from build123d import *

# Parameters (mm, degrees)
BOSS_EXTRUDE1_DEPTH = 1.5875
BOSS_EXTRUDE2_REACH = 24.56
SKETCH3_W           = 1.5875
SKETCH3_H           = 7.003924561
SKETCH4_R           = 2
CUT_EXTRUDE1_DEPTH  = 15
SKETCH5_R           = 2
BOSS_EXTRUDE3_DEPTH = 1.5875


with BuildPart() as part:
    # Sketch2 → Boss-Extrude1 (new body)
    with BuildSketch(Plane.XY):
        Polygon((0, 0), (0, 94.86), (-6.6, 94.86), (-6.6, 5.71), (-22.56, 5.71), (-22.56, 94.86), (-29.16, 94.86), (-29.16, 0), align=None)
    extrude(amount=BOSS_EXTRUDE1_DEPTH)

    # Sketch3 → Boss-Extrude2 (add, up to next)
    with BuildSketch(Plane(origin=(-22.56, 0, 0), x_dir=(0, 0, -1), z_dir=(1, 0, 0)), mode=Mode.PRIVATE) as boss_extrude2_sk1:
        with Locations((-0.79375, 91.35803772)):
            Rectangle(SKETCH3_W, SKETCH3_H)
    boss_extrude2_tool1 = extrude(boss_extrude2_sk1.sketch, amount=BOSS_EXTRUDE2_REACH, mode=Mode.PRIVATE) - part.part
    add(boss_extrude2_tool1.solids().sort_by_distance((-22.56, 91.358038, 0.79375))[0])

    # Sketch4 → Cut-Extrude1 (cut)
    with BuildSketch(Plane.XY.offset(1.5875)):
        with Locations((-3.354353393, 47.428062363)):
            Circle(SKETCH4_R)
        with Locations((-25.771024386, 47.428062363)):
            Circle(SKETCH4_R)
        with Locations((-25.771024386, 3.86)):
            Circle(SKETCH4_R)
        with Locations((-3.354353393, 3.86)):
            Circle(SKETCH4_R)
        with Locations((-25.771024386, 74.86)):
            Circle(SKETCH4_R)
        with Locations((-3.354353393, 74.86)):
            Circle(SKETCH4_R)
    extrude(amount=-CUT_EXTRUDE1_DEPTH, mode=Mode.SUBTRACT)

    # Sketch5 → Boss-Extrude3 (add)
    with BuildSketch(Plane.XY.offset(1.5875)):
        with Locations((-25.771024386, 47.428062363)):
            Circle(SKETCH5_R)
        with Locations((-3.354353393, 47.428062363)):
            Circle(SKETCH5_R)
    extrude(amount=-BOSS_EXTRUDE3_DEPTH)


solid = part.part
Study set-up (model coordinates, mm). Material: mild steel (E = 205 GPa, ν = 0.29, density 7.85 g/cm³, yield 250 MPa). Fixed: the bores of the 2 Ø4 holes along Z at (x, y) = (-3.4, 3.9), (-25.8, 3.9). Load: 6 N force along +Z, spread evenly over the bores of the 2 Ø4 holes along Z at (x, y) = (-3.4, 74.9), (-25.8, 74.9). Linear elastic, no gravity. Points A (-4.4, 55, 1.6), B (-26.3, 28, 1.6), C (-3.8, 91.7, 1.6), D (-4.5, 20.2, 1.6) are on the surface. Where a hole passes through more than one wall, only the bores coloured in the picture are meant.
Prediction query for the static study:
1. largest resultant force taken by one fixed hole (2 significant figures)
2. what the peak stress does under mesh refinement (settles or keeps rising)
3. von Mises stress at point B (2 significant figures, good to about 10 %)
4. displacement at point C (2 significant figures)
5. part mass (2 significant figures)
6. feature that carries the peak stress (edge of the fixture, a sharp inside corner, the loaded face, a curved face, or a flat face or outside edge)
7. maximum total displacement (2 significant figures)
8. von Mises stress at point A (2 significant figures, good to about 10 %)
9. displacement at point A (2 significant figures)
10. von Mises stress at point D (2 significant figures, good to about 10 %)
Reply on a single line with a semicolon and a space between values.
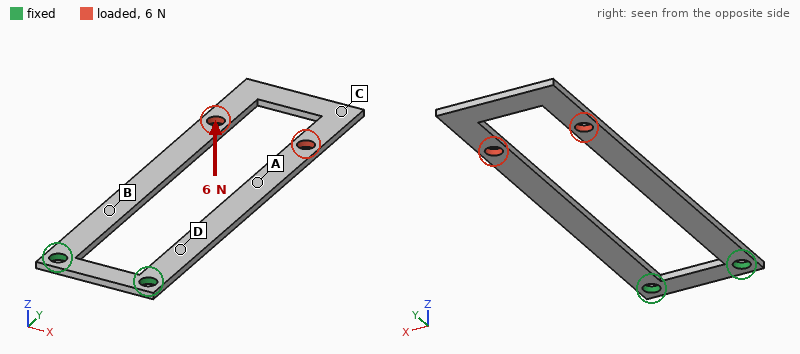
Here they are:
3.0 N; keeps rising; 51 MPa; 1.0 mm; 18 g; edge of the fixture; 1.1 mm; 22 MPa; 0.43 mm; 59 MPa
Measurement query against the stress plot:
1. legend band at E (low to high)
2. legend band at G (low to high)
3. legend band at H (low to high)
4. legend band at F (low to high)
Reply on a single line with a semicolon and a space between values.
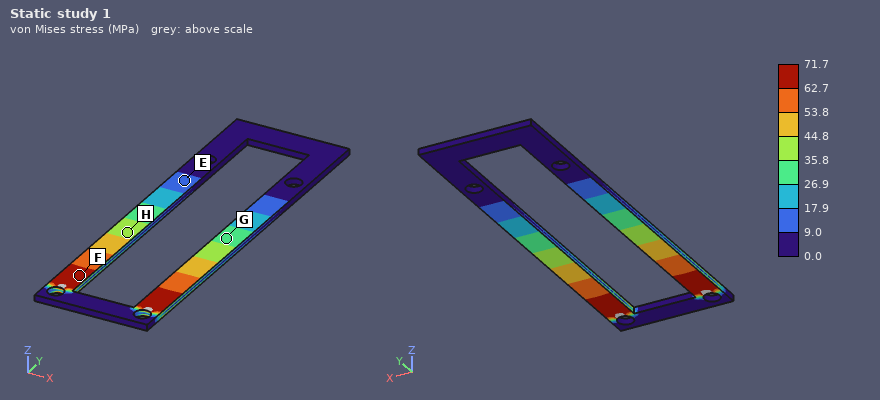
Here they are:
9.0 to 17.9 MPa; 26.9 to 35.8 MPa; 35.8 to 44.8 MPa; 62.7 to 71.7 MPa
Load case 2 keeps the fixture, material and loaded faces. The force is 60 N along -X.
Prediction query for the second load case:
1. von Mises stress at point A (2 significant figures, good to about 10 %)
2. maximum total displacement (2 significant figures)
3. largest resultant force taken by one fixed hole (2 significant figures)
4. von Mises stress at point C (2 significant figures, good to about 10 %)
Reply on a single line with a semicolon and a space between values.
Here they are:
15 MPa; 0.22 mm; 90 N; 27 MPa
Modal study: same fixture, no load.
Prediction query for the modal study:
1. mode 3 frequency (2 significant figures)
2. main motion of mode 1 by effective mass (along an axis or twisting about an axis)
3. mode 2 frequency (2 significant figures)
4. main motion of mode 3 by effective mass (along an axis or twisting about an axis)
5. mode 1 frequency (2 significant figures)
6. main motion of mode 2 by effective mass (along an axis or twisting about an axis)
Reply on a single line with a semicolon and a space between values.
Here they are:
920 Hz; along Z; 650 Hz; along Z; 140 Hz; twisting about Y
